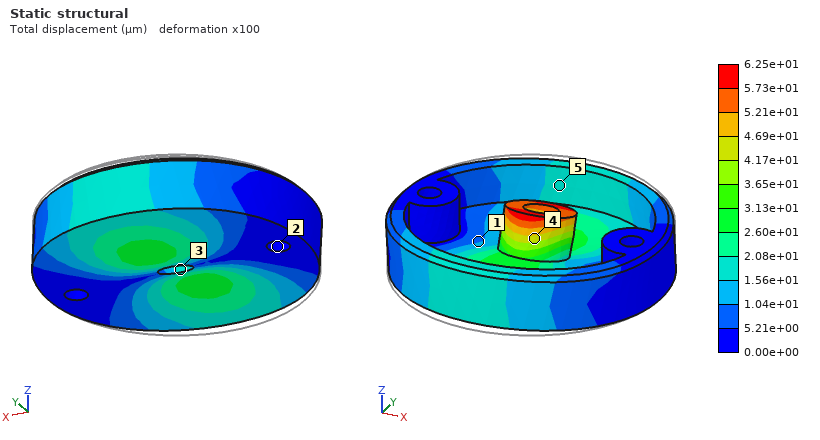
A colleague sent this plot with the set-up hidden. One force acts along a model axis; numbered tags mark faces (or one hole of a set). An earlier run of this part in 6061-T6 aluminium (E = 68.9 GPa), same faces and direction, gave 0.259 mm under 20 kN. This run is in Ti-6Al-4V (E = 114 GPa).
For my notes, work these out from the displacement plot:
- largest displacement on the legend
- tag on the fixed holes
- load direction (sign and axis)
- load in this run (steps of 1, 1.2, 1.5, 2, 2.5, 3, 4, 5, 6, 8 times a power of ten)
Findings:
6.25e+01 µm
2
+Y
8 kN
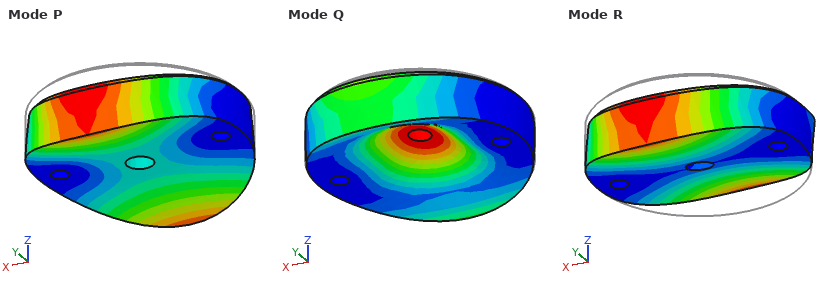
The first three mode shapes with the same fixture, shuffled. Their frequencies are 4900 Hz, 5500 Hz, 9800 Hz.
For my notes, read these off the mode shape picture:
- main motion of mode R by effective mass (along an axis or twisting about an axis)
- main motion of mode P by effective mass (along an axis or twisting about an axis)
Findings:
twisting about X
along Z
